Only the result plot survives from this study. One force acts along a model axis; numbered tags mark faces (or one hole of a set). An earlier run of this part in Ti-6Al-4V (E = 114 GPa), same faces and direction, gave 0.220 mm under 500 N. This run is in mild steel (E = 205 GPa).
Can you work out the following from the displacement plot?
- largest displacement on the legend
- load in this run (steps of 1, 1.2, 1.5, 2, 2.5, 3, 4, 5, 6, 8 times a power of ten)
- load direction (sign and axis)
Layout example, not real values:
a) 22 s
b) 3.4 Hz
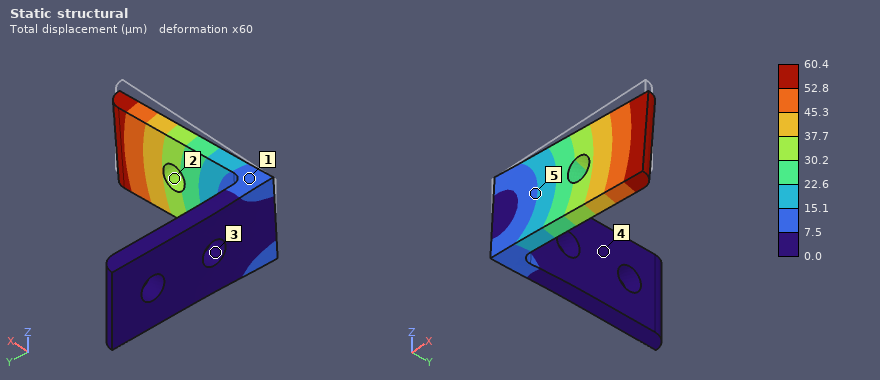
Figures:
a) 60.4 µm
b) 250 N
c) -Z
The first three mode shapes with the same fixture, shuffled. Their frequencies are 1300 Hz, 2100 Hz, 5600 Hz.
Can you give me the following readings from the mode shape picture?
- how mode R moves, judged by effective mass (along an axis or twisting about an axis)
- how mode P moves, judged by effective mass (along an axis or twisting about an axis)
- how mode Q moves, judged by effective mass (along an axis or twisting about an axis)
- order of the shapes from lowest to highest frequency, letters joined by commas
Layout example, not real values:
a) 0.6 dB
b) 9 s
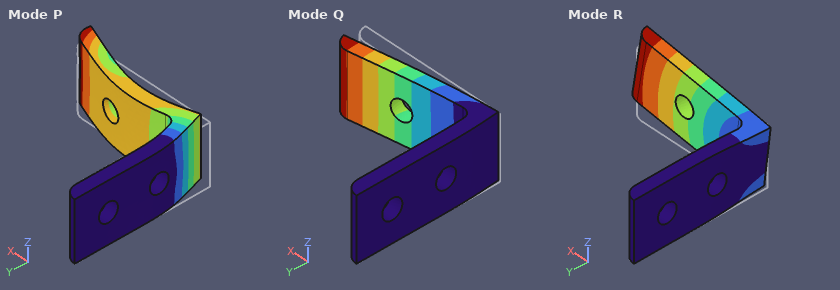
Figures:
a) along Z
b) along X
c) along Y
d) Q, R, P
